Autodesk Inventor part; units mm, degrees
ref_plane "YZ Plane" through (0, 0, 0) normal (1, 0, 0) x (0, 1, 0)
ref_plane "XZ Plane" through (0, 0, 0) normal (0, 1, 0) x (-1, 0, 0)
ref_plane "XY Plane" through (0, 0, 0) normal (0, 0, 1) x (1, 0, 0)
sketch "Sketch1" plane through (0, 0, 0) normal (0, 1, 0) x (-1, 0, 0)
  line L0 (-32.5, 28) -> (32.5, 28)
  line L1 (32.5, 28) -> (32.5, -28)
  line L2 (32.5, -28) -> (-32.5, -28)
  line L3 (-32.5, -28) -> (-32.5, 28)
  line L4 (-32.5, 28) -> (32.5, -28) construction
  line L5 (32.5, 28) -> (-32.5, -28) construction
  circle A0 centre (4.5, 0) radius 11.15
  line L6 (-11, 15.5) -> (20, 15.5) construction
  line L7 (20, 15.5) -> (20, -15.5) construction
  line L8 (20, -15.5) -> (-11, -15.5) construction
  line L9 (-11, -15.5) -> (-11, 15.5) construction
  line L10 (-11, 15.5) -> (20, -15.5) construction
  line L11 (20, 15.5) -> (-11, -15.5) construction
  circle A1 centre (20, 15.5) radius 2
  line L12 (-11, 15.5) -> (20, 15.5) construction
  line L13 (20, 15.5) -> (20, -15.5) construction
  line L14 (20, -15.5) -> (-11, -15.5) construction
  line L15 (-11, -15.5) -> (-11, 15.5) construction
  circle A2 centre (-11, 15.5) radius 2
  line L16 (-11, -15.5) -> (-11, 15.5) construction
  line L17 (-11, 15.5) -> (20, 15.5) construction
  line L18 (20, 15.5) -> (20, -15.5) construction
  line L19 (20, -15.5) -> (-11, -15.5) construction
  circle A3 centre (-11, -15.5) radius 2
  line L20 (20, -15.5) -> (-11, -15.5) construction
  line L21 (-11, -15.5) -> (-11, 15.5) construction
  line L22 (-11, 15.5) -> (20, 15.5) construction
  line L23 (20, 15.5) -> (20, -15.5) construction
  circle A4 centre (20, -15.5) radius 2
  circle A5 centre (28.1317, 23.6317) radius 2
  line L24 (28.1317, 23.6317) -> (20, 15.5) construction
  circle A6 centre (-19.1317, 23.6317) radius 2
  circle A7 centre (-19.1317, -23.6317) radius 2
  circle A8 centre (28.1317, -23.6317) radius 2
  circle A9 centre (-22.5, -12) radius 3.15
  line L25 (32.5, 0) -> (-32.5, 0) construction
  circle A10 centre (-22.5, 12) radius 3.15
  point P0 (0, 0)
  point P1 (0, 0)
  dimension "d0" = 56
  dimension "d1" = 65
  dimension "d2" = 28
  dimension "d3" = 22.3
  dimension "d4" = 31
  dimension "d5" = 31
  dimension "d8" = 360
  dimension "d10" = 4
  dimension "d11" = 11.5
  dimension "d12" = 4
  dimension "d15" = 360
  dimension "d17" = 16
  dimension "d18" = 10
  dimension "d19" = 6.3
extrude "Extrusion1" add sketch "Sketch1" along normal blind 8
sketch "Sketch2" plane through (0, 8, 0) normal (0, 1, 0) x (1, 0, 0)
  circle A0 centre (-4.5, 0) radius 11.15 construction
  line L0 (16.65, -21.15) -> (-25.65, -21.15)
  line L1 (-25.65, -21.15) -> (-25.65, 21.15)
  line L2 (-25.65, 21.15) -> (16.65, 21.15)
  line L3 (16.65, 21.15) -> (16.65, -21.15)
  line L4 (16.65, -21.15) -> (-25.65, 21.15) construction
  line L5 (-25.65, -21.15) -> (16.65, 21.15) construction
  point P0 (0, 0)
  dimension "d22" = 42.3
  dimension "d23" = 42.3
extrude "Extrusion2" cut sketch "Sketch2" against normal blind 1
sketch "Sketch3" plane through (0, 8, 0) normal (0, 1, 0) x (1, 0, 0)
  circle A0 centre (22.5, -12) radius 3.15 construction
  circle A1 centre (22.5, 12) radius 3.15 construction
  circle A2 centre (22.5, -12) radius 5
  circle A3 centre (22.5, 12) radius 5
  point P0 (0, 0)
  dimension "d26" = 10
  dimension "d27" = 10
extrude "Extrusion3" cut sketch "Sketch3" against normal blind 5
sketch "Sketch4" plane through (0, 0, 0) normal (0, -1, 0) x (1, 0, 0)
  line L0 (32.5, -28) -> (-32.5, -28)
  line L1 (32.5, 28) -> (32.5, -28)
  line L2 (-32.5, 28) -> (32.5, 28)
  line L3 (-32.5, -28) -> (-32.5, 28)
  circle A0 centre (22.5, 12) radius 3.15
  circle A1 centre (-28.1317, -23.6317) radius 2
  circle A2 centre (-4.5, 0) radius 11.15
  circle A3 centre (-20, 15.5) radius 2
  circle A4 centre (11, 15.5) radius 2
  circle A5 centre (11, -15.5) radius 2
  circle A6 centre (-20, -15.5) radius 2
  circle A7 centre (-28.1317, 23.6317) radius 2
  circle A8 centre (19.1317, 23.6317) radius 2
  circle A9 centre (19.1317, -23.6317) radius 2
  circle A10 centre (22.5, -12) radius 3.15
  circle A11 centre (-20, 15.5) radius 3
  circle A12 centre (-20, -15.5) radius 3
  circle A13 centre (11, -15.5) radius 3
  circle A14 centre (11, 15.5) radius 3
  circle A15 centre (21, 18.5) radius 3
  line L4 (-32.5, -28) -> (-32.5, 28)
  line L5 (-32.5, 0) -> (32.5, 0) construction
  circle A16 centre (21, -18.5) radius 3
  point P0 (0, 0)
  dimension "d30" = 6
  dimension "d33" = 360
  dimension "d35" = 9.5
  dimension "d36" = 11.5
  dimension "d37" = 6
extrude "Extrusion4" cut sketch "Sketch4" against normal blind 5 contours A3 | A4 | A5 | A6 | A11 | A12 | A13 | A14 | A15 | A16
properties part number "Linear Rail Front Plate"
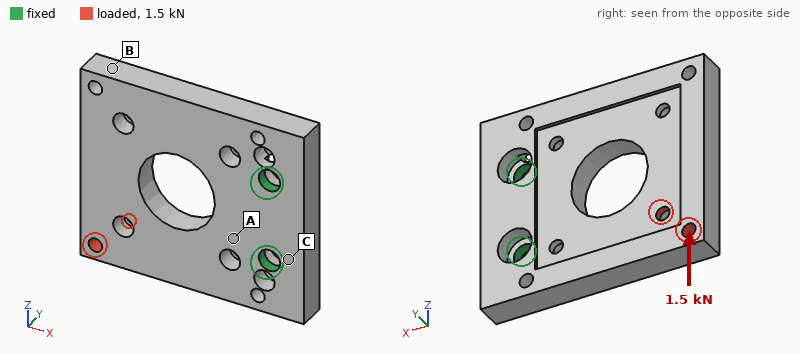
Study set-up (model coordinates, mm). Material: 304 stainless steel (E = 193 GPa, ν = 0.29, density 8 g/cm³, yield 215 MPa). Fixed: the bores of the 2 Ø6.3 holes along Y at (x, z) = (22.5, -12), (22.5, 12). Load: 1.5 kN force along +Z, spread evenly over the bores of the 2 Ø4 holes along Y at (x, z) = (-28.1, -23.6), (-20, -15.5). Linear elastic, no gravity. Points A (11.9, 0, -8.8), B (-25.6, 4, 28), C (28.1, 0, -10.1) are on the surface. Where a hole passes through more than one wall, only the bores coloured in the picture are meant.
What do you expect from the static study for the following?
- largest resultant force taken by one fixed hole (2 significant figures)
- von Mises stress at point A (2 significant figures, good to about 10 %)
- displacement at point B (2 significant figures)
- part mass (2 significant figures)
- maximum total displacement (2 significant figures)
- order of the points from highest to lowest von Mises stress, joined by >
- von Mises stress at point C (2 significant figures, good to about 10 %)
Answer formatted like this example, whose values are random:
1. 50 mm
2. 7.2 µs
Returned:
1. 2.8 kN
2. 20 MPa
3. 22 µm
4. 180 g
5. 27 µm
6. C > A > B
7. 36 MPa
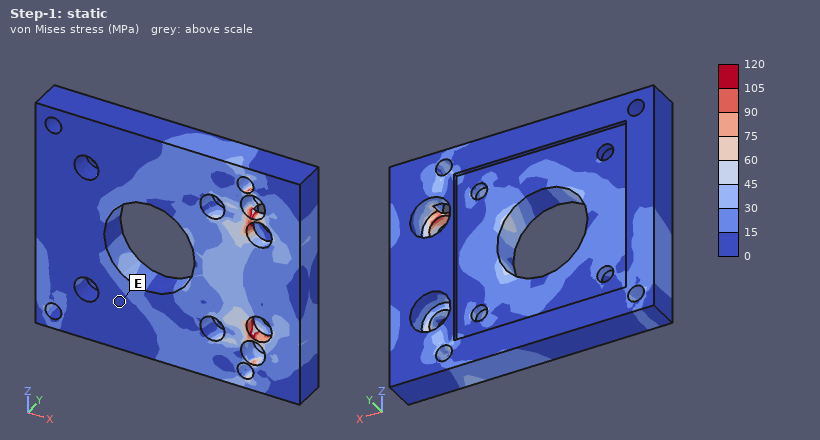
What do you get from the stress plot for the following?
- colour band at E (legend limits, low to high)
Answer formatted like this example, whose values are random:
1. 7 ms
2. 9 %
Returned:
1. 0 to 15 MPa
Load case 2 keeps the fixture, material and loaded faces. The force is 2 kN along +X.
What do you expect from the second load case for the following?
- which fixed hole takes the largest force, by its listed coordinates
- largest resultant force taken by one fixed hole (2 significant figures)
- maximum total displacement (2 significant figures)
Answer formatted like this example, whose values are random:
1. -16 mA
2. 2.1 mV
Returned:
1. (22.5, -12)
2. 2.6 kN
3. 35 µm
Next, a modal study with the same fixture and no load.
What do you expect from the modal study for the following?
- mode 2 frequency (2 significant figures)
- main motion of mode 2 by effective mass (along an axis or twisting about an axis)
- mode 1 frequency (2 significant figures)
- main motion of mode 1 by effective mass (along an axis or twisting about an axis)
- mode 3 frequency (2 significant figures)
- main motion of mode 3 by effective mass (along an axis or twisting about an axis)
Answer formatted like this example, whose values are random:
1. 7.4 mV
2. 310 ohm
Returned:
1. 3100 Hz
2. twisting about X
3. 1300 Hz
4. along Y
5. 4900 Hz
6. along Z
